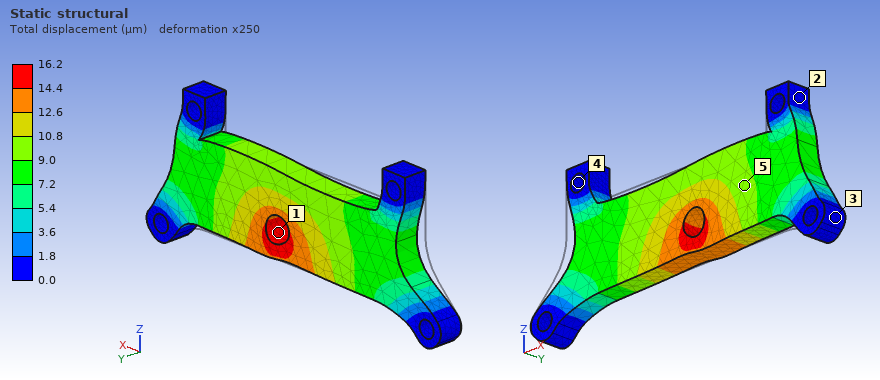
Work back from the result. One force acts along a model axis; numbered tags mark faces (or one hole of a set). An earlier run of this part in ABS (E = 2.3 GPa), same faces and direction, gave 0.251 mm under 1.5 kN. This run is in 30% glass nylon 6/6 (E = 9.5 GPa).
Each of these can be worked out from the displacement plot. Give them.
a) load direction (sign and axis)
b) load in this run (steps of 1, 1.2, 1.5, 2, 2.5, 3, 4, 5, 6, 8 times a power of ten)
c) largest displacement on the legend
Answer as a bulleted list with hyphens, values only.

- +X
- 400 N
- 16.2 µm
